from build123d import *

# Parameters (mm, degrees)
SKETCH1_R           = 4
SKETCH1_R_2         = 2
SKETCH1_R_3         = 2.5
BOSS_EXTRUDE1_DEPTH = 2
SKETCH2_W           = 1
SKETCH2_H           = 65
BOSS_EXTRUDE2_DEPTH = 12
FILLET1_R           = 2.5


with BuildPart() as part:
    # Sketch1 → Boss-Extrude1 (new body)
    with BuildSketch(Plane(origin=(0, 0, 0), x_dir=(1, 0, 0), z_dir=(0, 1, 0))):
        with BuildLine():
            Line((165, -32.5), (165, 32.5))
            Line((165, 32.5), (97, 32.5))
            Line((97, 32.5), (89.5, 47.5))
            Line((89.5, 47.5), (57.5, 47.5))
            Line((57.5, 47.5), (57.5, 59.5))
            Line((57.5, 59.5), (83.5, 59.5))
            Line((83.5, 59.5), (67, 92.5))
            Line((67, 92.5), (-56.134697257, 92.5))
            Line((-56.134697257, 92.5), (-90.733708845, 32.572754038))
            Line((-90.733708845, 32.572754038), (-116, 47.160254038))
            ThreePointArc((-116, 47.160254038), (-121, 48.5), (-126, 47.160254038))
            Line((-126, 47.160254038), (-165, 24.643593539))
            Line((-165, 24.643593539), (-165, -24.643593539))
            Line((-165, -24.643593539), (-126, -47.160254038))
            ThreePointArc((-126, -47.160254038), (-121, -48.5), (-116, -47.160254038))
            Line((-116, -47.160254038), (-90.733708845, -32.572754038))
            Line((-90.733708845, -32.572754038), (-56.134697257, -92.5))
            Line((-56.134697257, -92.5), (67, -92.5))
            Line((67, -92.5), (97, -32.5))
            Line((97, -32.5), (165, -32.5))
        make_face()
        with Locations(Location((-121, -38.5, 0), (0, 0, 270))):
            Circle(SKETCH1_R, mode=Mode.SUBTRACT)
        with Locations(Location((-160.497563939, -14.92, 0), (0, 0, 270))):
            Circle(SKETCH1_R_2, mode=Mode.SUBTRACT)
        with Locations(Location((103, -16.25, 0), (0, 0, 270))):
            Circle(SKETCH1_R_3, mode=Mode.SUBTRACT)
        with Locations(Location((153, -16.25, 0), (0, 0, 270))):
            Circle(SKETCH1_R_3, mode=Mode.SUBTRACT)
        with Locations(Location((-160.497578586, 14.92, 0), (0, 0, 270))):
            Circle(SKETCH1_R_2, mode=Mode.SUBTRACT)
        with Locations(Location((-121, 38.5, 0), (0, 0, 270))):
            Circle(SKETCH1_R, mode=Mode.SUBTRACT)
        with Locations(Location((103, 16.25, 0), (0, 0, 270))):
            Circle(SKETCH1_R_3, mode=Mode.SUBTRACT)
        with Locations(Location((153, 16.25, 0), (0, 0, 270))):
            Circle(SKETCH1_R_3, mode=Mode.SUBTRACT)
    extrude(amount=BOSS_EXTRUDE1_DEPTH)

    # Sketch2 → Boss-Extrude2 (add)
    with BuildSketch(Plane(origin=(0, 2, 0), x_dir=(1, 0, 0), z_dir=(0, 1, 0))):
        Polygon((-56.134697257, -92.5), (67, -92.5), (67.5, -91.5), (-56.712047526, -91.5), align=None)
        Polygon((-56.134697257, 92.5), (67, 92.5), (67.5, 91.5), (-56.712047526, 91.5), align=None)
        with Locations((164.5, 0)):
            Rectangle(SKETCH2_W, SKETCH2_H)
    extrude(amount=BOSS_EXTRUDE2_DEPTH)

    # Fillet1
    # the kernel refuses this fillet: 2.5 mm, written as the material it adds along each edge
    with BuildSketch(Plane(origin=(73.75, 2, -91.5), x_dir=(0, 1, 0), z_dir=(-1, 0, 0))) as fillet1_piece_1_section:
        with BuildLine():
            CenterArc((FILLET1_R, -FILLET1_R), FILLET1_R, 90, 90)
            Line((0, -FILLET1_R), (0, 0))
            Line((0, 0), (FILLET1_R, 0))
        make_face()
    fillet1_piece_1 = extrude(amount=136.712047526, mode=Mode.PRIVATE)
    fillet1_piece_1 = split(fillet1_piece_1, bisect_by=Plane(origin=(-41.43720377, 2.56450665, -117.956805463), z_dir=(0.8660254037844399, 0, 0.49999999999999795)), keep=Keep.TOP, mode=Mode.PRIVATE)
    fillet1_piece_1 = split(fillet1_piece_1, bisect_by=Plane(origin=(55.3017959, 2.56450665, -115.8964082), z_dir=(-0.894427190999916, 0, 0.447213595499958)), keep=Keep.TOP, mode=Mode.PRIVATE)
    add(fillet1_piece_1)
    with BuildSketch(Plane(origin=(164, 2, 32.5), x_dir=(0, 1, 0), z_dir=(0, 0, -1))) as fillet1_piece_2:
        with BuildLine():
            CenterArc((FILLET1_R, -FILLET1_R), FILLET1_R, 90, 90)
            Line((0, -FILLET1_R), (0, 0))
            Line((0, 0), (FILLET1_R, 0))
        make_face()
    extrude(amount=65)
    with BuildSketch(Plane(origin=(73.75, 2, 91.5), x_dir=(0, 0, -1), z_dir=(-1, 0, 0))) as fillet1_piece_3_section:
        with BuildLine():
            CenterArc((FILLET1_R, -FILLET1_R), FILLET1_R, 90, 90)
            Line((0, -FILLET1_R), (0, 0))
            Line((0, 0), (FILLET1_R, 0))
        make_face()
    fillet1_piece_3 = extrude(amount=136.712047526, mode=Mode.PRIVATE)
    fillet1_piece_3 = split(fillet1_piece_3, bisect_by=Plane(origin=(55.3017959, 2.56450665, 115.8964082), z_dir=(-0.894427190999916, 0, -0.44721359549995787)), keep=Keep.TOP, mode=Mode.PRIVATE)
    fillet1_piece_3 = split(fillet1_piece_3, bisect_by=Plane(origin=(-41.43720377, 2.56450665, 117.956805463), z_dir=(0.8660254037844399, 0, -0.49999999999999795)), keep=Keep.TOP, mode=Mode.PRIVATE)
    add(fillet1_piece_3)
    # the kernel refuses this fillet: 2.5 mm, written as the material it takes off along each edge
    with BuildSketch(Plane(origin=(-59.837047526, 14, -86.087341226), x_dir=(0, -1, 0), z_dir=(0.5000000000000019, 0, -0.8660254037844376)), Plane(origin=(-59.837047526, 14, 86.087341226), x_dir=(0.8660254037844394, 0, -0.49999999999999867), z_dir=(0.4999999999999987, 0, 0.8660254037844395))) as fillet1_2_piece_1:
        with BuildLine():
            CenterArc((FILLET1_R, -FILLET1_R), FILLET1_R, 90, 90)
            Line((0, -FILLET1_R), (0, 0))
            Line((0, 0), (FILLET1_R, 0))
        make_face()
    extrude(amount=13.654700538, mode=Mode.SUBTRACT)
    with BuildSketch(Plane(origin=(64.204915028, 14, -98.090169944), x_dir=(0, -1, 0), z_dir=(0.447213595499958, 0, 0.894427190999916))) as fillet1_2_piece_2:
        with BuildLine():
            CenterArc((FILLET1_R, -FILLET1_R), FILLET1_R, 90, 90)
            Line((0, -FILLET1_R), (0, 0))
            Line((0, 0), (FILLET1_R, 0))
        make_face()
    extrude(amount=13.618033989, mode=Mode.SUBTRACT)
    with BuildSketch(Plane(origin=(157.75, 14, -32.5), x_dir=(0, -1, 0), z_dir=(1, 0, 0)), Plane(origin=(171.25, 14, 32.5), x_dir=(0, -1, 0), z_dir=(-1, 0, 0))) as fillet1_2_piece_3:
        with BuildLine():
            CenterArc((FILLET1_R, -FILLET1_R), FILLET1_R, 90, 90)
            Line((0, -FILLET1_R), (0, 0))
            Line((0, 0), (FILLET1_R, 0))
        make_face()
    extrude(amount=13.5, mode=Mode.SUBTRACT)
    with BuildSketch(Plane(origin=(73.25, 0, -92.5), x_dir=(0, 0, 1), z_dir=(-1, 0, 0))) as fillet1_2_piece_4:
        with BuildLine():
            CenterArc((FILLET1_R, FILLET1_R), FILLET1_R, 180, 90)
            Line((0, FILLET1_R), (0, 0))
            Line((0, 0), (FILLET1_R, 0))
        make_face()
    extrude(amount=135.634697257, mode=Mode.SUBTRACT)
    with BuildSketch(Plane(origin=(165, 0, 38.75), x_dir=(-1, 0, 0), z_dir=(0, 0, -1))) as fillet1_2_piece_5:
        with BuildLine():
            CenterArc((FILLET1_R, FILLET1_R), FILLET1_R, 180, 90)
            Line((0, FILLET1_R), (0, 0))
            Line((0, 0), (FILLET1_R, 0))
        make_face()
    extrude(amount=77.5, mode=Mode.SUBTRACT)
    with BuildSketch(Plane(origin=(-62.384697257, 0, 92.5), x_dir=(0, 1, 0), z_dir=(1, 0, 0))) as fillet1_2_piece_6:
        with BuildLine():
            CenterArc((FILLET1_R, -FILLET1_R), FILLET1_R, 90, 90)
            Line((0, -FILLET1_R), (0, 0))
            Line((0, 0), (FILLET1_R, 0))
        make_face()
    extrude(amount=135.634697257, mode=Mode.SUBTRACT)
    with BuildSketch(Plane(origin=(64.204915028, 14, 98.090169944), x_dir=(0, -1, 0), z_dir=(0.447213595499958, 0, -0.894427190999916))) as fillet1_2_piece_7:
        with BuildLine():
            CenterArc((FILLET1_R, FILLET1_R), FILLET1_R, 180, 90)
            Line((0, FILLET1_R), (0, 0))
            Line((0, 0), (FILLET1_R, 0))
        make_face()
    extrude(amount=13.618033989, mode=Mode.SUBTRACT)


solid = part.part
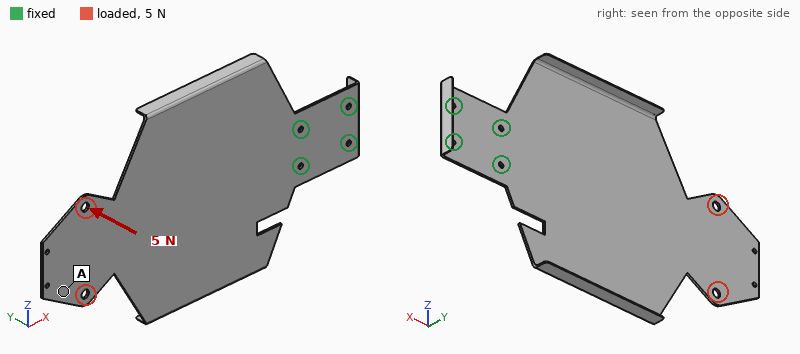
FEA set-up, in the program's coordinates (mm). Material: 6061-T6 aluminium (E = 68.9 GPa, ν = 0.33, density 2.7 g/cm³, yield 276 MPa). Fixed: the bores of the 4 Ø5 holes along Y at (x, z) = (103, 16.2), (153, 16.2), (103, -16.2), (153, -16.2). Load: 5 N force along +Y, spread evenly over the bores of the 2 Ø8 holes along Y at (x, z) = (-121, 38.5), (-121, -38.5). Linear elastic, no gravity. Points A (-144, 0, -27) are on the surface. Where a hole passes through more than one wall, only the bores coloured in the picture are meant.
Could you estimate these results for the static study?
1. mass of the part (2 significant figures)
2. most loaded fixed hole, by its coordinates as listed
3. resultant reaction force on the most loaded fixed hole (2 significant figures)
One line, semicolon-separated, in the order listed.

230 g; (103, 16.2); 4.4 N
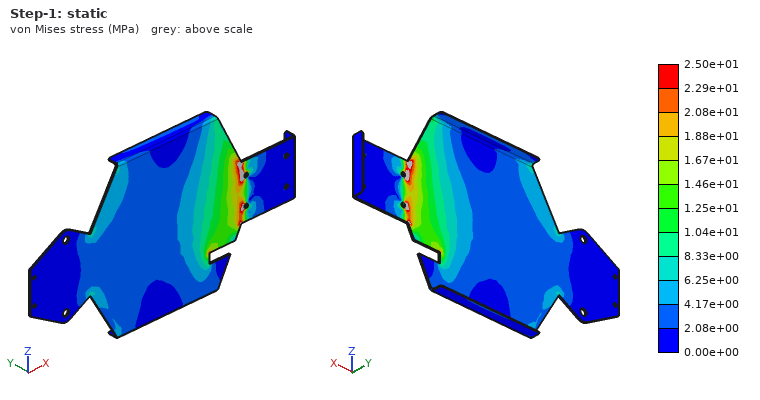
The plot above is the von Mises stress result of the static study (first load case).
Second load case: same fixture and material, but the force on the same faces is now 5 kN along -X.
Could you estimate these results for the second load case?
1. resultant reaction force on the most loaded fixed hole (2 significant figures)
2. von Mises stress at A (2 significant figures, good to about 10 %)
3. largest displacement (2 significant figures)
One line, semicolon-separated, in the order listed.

2.1 kN; 22 MPa; 0.12 mm
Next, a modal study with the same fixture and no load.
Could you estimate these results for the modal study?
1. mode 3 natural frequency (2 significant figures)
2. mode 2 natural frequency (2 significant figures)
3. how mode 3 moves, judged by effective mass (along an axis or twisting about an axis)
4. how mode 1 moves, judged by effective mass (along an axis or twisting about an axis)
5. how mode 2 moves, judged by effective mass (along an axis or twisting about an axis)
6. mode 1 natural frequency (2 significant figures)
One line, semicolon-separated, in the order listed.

130 Hz; 75 Hz; along Y; along Y; twisting about X; 25 Hz
